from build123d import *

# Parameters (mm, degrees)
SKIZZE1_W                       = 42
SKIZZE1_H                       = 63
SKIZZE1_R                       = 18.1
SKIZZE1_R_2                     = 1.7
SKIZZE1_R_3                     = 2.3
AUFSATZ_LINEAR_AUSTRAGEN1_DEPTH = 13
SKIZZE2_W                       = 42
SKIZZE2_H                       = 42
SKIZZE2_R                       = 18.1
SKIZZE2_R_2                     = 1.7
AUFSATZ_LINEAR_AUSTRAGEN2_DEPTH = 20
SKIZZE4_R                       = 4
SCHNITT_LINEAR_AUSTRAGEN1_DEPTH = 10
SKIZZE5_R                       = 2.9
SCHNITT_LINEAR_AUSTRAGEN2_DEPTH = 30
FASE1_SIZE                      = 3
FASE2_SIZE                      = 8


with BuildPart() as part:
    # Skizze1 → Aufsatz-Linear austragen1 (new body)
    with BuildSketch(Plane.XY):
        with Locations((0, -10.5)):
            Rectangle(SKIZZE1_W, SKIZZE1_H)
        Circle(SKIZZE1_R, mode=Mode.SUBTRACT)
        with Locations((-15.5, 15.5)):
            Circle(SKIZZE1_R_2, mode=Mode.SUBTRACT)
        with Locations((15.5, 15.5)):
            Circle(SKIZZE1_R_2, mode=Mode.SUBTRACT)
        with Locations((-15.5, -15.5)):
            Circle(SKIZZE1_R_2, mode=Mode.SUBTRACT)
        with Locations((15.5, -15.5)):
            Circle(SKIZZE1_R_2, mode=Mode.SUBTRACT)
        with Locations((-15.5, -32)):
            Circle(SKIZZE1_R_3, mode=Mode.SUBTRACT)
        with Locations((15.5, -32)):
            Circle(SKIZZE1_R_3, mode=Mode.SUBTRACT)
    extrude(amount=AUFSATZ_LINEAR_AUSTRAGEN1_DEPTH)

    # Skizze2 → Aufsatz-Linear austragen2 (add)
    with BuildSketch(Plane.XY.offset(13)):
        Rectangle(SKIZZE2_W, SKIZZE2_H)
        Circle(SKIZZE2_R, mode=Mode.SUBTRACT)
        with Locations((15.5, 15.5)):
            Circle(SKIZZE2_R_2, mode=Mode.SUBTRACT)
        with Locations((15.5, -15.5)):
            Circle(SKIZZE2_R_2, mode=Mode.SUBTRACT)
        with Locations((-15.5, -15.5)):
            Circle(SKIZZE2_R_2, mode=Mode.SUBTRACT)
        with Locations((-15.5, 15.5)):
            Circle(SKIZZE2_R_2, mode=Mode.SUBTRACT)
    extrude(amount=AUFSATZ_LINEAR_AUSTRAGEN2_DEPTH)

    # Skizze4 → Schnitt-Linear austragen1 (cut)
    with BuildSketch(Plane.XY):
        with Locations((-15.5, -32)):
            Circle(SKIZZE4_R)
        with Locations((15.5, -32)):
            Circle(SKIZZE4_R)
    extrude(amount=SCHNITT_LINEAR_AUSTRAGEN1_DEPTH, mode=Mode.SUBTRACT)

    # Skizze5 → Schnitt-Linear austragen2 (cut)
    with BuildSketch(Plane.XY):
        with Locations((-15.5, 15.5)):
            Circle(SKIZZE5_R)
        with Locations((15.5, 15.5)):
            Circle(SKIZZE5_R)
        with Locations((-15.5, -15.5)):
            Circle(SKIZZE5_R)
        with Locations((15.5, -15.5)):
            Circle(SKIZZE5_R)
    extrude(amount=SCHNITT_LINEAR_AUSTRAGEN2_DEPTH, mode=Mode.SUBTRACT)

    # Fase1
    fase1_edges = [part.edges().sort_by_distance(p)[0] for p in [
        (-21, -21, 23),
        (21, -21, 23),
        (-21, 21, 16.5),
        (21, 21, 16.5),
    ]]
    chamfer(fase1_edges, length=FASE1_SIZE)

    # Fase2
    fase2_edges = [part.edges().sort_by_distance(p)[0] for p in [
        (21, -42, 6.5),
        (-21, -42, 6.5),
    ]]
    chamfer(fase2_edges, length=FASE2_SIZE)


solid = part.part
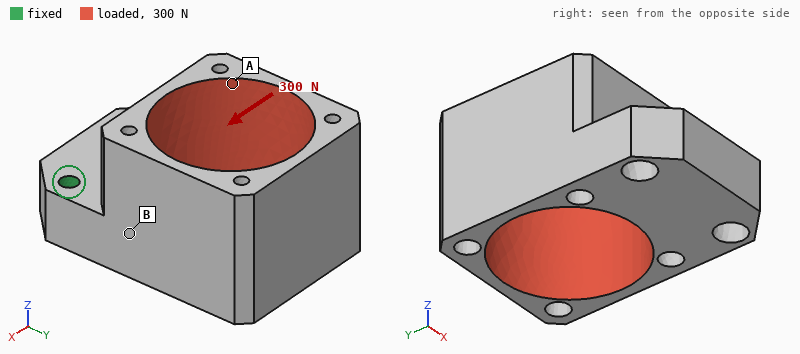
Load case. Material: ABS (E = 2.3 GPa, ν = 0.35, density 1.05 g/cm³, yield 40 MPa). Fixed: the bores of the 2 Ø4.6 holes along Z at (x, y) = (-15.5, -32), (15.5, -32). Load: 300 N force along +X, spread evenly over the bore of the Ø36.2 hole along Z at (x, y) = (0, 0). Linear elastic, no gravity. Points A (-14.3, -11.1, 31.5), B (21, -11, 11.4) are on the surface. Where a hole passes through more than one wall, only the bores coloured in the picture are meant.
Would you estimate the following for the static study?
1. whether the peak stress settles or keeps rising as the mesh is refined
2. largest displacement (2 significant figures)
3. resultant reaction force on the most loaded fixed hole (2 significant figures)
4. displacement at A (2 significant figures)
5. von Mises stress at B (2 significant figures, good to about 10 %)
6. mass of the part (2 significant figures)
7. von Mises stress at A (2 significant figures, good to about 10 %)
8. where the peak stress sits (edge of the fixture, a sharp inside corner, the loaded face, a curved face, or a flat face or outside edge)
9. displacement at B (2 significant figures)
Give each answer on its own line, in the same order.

keeps rising
0.53 mm
330 N
0.17 mm
6.6 MPa
32 g
3.5 MPa
edge of the fixture
0.14 mm
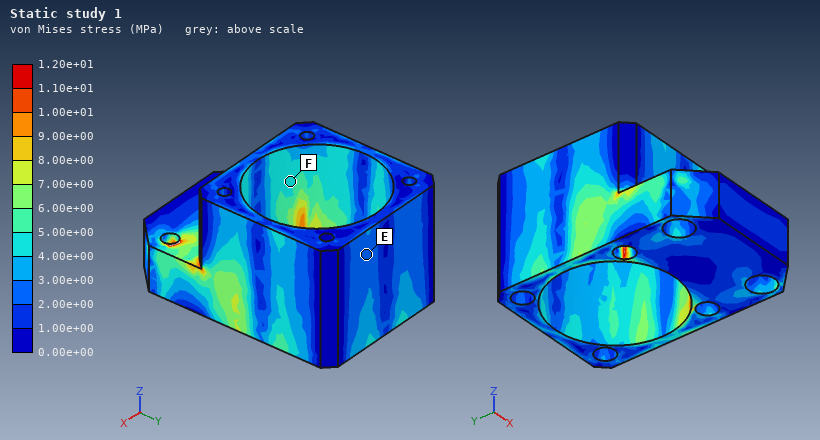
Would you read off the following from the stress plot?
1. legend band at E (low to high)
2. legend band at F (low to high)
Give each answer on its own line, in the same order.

2.00e+00 to 3.00e+00 MPa
4.00e+00 to 5.00e+00 MPa
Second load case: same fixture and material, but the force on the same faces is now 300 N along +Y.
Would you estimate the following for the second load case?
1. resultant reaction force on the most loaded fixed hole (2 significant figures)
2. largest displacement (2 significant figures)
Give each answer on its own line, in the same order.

150 N
0.77 mm
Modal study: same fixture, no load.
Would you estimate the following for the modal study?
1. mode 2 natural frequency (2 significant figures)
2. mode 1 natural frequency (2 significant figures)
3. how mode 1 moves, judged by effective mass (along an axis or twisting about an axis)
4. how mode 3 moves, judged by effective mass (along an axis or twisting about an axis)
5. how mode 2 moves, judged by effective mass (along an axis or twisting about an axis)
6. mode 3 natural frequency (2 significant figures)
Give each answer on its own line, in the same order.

920 Hz
360 Hz
along Z
twisting about Y
along X
1300 Hz
